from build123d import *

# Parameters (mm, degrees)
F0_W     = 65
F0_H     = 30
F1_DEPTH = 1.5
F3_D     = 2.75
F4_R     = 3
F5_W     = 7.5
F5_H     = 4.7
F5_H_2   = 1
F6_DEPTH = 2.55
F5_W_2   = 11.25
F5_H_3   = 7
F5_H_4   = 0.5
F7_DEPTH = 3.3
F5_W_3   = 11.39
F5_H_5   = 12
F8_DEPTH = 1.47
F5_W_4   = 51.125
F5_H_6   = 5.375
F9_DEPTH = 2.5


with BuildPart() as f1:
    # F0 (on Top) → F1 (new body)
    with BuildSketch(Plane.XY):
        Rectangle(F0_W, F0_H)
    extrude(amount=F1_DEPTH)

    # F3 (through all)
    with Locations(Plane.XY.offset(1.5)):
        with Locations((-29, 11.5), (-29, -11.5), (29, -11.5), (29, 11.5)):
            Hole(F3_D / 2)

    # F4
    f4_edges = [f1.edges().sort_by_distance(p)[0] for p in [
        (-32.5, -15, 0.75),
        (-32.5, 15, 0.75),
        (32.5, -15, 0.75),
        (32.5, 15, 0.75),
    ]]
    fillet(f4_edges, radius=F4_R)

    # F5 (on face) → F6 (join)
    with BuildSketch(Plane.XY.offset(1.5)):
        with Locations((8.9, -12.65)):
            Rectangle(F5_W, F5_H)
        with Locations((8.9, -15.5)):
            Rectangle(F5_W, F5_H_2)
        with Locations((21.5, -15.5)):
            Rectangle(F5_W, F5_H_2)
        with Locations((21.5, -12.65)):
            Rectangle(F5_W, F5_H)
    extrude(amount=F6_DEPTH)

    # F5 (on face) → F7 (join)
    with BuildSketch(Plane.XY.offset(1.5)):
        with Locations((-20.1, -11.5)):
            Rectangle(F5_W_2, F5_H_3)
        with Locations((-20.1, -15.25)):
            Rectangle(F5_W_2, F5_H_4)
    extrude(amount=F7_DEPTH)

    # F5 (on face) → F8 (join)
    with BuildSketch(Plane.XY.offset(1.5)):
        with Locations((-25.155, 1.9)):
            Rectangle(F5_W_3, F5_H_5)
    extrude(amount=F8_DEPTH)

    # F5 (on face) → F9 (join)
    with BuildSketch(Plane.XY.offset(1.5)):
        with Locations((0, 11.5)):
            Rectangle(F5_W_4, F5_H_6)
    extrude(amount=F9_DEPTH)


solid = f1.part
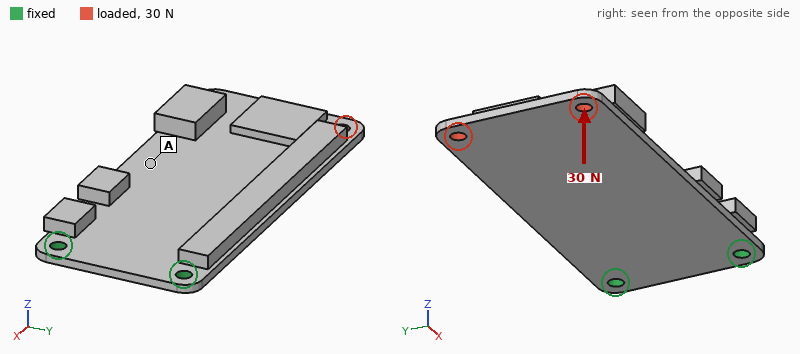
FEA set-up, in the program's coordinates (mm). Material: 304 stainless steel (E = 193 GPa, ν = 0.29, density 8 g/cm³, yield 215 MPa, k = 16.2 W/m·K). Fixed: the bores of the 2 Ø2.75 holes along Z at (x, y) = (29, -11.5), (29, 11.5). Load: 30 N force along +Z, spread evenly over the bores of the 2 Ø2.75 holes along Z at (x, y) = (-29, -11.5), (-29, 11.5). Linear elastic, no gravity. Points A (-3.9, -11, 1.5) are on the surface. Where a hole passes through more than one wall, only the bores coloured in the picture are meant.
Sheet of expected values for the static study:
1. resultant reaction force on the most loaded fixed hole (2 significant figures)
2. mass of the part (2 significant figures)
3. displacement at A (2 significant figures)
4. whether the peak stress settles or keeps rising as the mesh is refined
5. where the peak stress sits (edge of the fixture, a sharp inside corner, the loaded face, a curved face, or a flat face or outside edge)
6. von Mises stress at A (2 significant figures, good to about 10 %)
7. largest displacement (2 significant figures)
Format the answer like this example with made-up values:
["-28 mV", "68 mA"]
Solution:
["43 N", "34 g", "0.23 mm", "keeps rising", "edge of the fixture", "25 MPa", "0.55 mm"]
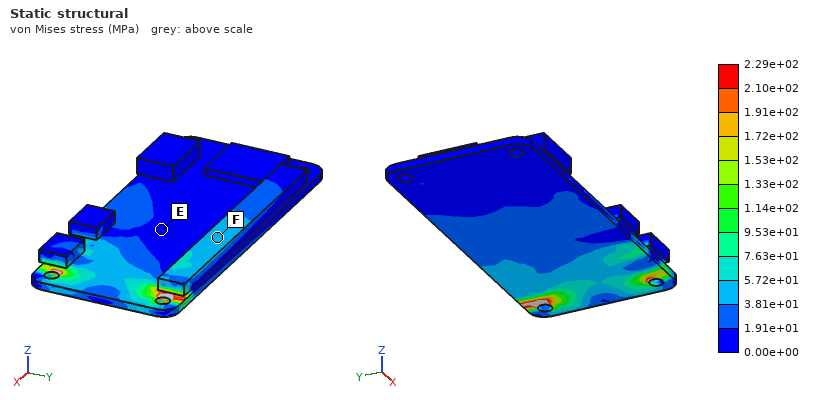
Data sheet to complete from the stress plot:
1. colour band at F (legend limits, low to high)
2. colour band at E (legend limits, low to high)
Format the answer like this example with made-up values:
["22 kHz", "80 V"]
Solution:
["3.81e+01 to 5.72e+01 MPa", "0.00e+00 to 1.91e+01 MPa"]
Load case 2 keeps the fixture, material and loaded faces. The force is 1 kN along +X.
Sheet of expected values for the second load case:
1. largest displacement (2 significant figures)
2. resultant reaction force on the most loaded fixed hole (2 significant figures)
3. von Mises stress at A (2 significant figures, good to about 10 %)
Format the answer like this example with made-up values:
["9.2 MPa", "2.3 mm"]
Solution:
["69 µm", "510 N", "19 MPa"]
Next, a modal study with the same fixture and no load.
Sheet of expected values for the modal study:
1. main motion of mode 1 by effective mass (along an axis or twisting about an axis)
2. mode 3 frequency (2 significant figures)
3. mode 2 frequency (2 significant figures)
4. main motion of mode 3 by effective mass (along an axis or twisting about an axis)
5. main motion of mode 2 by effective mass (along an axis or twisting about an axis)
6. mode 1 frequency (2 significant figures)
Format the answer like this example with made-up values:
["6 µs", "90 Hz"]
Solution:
["along Z", "2900 Hz", "1600 Hz", "along Z", "twisting about X", "360 Hz"]
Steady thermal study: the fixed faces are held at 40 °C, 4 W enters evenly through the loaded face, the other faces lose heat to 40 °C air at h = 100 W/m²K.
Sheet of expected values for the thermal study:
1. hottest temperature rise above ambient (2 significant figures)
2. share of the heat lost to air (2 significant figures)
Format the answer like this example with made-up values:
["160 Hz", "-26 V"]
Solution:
["61 K", "99 %"]
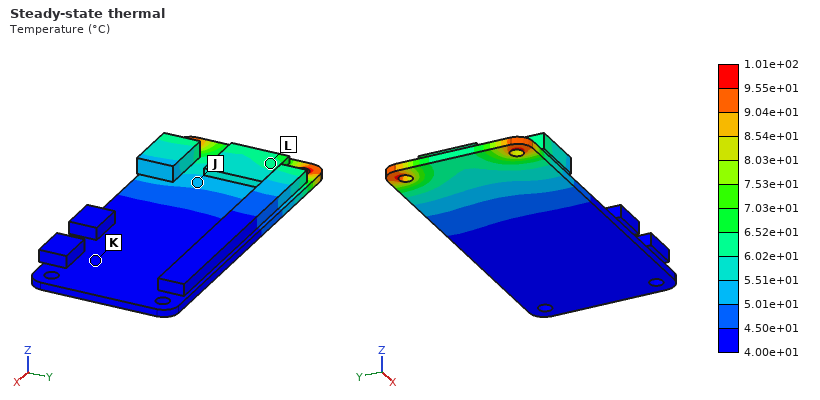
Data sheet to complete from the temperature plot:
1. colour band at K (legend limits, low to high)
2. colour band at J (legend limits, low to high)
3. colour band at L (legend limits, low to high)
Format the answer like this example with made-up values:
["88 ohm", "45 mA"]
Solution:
["4.00e+01 to 4.50e+01 °C", "5.01e+01 to 5.51e+01 °C", "6.02e+01 to 6.52e+01 °C"]
